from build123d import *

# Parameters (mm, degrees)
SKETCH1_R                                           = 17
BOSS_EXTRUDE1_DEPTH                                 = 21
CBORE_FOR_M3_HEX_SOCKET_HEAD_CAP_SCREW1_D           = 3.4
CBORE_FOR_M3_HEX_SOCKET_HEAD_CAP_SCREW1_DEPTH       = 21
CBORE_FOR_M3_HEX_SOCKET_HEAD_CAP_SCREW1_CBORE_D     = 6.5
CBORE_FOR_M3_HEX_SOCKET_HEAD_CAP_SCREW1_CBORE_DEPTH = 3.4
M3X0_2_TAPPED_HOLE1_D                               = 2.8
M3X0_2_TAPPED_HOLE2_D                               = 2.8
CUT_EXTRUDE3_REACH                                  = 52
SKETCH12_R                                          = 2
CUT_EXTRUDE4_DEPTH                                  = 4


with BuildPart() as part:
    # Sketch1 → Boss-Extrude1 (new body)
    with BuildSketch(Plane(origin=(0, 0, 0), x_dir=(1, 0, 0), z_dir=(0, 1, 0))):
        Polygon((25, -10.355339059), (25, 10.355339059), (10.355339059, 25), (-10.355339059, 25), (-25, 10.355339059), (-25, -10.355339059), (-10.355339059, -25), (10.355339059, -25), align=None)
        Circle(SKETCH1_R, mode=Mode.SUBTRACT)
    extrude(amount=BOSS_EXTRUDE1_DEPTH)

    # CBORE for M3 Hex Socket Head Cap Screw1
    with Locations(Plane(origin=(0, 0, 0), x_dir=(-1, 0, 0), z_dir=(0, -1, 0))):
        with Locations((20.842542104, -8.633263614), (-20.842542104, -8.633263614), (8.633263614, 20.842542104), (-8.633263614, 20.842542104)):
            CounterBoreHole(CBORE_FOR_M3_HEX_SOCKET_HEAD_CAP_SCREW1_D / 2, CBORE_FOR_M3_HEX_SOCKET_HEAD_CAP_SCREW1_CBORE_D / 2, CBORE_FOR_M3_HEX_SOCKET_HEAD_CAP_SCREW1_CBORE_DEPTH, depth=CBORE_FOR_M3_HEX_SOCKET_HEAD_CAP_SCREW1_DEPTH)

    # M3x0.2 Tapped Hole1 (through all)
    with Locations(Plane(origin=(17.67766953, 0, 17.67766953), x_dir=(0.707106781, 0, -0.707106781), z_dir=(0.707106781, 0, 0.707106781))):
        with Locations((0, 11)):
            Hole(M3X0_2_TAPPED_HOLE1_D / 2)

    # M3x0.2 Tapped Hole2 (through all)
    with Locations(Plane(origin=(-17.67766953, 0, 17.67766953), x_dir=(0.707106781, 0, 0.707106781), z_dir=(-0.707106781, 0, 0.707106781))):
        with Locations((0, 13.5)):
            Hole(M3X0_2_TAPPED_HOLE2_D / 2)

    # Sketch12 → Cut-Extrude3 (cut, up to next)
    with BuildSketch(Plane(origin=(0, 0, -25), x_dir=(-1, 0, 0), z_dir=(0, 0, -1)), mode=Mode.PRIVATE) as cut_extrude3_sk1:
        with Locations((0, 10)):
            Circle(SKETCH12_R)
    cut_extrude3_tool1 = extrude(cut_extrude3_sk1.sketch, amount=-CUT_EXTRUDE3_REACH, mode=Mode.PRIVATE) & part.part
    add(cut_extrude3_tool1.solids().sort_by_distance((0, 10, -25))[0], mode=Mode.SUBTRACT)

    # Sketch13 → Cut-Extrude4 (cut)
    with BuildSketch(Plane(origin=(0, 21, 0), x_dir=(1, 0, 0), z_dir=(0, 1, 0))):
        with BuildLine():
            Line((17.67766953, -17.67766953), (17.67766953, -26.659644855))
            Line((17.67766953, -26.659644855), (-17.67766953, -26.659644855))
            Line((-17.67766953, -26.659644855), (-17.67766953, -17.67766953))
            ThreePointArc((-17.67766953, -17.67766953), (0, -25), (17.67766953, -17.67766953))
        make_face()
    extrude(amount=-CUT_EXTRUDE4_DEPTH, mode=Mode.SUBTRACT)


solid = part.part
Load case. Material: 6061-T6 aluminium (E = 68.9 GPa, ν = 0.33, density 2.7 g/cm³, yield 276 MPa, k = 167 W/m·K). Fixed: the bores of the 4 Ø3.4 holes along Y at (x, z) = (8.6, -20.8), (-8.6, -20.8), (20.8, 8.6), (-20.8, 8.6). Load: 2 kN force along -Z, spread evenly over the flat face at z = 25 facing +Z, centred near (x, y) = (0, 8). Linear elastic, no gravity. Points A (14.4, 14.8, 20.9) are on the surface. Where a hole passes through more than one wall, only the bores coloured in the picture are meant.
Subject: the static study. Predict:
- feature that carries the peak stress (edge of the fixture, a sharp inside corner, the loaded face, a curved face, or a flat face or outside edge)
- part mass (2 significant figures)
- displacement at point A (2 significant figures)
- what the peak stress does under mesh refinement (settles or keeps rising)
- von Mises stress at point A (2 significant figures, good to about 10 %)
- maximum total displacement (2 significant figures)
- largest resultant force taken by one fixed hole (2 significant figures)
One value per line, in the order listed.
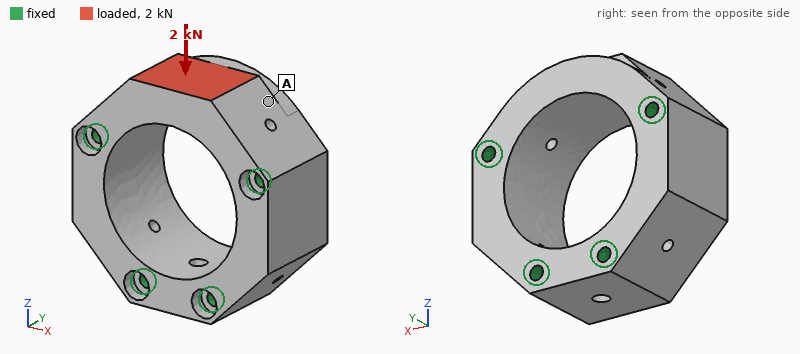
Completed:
edge of the fixture
62 g
1.9 µm
keeps rising
5.3 MPa
8.8 µm
1.3 kN
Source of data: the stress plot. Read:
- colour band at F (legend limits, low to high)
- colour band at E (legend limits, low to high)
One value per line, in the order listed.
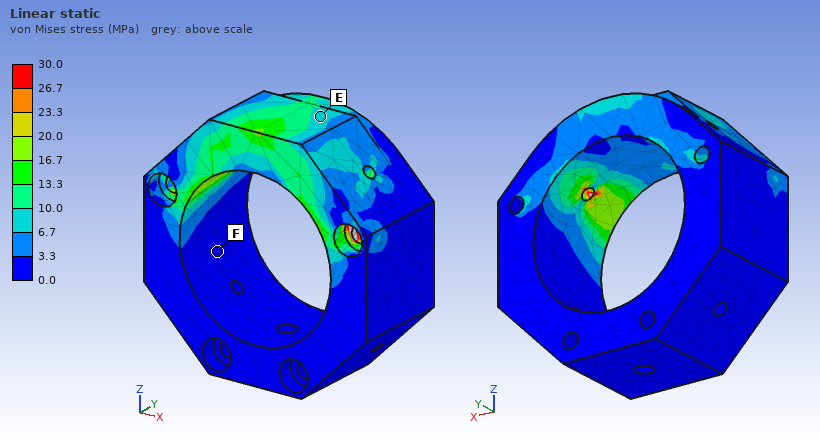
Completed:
0.0 to 3.3 MPa
6.7 to 10.0 MPa
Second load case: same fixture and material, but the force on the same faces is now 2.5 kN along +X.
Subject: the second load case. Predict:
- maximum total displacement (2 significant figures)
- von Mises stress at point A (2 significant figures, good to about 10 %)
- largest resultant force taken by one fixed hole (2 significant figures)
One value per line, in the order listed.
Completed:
5.3 µm
7.1 MPa
1.5 kN
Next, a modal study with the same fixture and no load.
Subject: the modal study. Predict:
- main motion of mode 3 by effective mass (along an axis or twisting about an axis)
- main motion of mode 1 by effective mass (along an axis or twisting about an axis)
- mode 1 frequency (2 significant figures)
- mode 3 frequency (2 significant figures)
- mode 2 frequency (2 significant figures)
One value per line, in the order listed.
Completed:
along Z
along Y
18 kHz
29 kHz
27 kHz
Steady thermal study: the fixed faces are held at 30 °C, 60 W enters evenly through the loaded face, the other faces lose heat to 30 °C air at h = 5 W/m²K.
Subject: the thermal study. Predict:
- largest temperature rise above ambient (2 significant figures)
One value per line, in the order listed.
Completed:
25 K
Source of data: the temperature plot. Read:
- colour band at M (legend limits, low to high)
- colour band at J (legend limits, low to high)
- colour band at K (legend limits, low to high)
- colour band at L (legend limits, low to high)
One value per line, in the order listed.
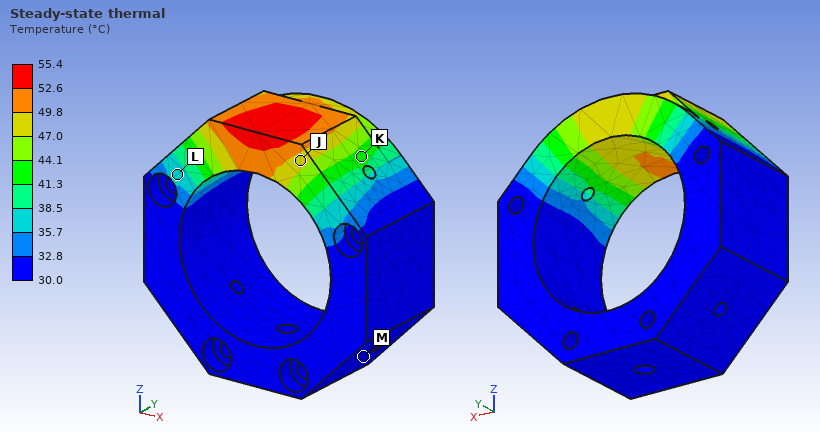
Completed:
30.0 to 32.8 °C
47.0 to 49.8 °C
41.3 to 44.1 °C
35.7 to 38.5 °C
